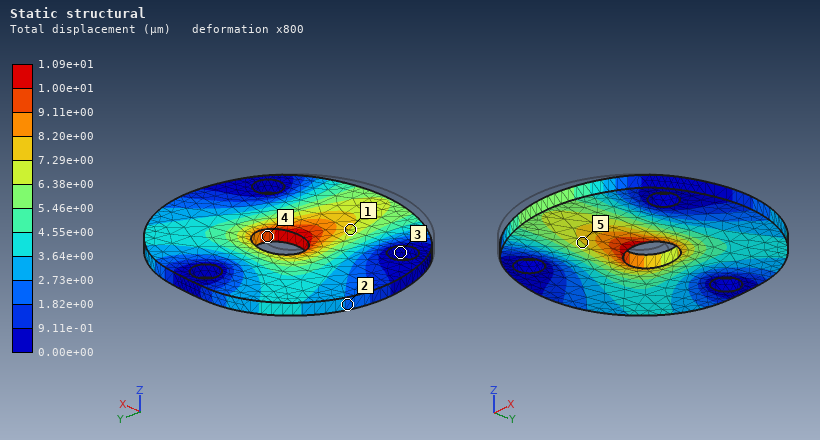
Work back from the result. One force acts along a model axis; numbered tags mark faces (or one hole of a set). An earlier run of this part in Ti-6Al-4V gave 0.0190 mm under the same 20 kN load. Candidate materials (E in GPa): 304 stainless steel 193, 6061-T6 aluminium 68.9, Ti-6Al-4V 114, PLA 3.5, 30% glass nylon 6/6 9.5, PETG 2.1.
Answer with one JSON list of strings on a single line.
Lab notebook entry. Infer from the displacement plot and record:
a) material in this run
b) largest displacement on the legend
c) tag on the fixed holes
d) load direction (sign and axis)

["304 stainless steel", "1.09e+01 µm", "3", "+Y"]
